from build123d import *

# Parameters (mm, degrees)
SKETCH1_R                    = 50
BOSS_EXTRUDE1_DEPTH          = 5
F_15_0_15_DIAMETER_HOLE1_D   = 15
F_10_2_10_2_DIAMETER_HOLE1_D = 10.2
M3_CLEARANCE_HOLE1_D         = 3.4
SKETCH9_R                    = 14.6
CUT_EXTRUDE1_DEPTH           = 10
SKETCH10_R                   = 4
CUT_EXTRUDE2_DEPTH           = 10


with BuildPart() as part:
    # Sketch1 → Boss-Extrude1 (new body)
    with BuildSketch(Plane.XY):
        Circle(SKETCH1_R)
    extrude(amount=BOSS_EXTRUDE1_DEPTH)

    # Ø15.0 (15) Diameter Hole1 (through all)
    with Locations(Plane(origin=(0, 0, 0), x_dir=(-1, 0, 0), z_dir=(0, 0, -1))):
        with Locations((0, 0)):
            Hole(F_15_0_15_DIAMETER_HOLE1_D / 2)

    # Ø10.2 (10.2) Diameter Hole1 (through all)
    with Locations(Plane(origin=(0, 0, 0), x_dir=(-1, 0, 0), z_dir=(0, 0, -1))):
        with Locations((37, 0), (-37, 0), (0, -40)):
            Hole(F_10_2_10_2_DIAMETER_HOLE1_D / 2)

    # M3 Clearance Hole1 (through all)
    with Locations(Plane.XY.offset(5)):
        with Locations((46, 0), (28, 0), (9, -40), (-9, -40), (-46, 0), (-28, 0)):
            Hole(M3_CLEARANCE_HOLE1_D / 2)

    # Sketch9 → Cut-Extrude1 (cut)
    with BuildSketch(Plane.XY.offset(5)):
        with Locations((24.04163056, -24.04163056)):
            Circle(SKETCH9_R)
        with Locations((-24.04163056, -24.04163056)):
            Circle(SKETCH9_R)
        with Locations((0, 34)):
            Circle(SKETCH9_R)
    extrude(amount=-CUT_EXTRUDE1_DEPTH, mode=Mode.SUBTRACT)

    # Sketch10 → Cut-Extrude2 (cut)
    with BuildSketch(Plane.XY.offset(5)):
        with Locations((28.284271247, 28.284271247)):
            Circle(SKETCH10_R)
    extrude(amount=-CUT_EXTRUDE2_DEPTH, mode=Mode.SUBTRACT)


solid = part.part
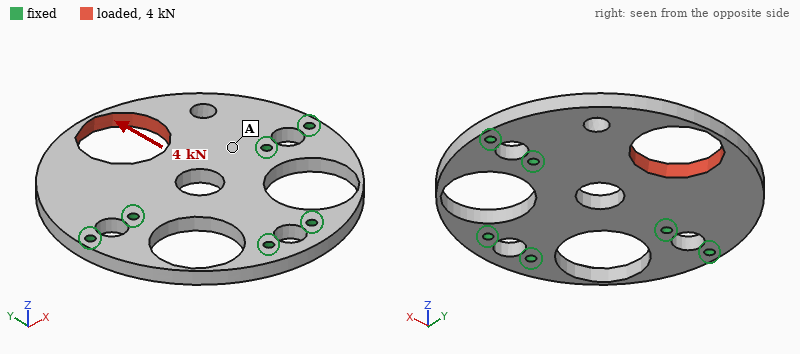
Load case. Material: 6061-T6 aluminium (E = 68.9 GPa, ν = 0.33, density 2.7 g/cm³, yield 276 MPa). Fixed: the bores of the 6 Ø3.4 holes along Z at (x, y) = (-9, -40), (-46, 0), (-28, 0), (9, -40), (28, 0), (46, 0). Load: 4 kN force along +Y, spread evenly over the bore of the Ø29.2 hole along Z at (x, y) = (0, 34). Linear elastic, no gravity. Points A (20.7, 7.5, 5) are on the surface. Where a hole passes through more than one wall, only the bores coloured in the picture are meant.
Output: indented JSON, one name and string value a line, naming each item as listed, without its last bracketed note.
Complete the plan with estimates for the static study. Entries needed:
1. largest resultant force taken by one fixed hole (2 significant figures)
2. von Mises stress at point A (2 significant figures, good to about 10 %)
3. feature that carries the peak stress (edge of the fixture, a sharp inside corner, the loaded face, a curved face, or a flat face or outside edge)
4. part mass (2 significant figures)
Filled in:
{
  "largest resultant force taken by one fixed hole": "1.4 kN",
  "von Mises stress at point A": "16 MPa",
  "feature that carries the peak stress": "a curved face",
  "part mass": "72 g"
}
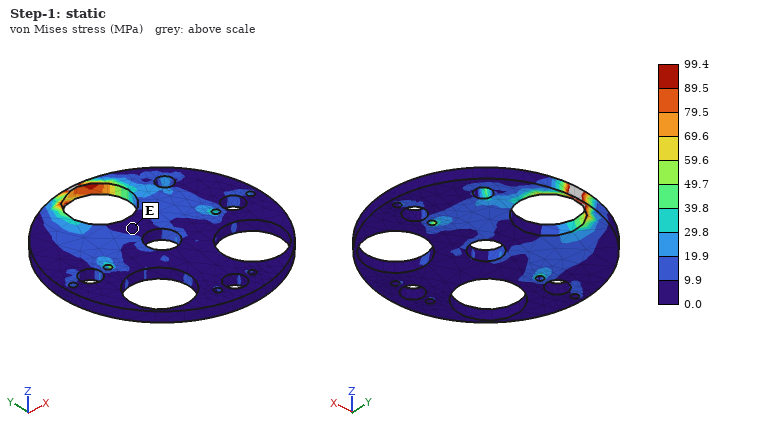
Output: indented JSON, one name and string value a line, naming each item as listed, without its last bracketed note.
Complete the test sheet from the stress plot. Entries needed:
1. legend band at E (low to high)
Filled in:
{
  "legend band at E": "0.0 to 9.9 MPa"
}
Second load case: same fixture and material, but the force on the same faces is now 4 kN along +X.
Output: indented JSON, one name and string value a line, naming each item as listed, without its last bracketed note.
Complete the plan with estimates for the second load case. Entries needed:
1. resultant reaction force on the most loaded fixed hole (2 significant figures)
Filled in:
{
  "resultant reaction force on the most loaded fixed hole": "1.6 kN"
}
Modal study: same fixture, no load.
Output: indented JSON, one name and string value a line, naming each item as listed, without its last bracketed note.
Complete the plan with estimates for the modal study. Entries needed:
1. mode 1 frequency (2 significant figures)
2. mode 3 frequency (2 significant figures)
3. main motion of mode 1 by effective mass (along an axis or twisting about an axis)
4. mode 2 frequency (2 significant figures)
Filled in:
{
  "mode 1 frequency": "2200 Hz",
  "mode 3 frequency": "6900 Hz",
  "main motion of mode 1 by effective mass": "along Z",
  "mode 2 frequency": "3700 Hz"
}
